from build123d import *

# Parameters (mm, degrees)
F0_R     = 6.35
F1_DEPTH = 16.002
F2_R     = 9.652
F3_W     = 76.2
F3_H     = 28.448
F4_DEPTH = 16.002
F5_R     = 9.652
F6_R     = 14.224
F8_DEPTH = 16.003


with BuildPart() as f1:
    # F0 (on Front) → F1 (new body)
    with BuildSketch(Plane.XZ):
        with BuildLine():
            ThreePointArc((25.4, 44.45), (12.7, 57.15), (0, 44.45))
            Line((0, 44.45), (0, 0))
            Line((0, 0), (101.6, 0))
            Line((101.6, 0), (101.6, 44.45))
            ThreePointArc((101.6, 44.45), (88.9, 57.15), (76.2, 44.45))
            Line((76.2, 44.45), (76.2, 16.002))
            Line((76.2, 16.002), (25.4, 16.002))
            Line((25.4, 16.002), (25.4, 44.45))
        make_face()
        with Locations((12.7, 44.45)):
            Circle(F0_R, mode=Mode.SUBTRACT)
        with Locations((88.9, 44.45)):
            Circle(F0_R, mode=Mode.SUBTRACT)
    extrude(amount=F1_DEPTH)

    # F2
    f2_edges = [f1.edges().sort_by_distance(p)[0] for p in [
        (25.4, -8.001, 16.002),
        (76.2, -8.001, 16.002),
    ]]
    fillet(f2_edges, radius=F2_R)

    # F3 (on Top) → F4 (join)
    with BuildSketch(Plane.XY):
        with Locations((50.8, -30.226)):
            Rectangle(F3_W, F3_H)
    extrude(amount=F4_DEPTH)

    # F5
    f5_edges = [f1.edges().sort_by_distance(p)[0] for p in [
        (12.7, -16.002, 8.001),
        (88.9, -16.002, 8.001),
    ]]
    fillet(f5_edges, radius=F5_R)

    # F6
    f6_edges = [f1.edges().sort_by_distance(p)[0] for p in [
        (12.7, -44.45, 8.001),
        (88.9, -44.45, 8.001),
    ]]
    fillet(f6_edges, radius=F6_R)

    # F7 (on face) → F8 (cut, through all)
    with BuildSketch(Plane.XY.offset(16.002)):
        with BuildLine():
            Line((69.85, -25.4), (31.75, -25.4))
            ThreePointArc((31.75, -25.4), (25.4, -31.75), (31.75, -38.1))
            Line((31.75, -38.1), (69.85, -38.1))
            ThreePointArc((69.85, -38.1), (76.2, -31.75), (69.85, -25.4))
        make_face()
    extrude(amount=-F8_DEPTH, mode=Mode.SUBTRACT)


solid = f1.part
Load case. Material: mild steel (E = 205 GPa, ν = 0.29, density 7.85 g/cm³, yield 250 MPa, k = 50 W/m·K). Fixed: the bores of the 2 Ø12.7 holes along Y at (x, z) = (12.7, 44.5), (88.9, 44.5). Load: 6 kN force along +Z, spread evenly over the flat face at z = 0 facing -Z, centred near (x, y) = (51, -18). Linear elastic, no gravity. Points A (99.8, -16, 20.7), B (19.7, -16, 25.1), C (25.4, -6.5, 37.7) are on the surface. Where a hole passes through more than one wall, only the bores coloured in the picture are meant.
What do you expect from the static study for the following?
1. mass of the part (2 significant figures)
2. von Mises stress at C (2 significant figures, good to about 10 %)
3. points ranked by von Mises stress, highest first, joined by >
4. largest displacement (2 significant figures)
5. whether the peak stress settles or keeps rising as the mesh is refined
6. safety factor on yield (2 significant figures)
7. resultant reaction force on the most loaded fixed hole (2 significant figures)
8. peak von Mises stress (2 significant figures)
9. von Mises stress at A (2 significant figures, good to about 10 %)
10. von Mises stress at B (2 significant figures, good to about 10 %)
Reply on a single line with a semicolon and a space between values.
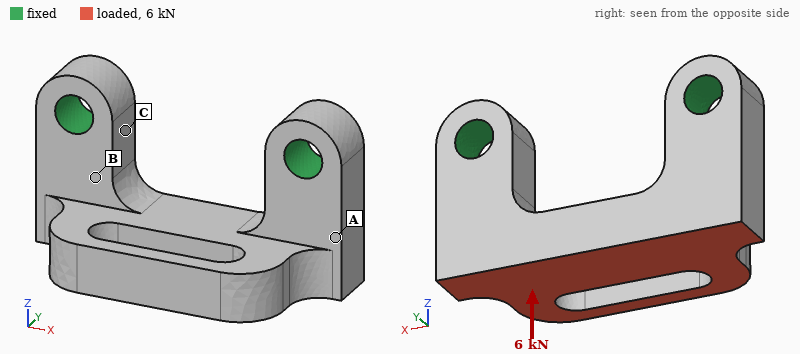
610 g; 8.0 MPa; B > A > C; 33 µm; settles; 4.0; 3.1 kN; 63 MPa; 21 MPa; 38 MPa
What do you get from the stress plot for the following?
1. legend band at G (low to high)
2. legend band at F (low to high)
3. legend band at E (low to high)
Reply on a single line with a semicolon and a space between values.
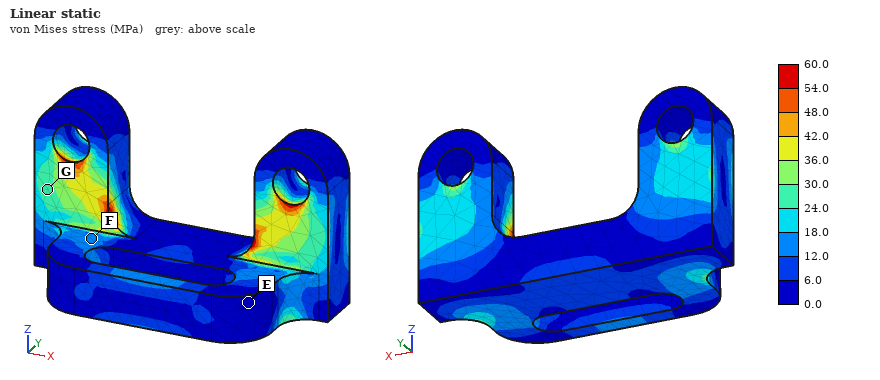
24.0 to 30.0 MPa; 12.0 to 18.0 MPa; 0.0 to 6.0 MPa
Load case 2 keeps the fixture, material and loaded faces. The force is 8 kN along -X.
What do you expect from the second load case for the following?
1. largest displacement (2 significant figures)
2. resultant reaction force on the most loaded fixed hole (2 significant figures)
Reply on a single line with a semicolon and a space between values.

17 µm; 4.8 kN
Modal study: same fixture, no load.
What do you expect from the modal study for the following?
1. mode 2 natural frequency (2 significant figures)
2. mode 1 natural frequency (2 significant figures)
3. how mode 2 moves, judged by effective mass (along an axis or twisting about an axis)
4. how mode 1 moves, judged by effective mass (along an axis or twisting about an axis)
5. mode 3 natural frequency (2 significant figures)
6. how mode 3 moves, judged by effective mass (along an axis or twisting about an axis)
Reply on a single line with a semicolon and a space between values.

5600 Hz; 3200 Hz; along X; along Y; 7200 Hz; along X
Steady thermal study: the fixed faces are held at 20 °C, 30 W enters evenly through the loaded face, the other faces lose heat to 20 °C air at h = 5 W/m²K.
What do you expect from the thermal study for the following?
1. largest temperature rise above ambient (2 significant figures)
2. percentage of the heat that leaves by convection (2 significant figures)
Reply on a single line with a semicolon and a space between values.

34 K; 4.3 %
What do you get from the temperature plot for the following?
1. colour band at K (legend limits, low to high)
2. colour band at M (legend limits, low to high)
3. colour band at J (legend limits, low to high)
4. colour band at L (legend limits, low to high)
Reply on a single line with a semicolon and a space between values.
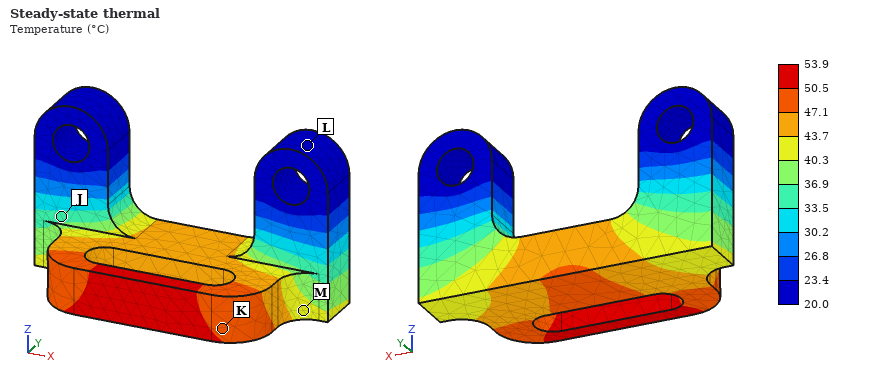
47.1 to 50.5 °C; 40.3 to 43.7 °C; 33.5 to 36.9 °C; 20.0 to 23.4 °C
